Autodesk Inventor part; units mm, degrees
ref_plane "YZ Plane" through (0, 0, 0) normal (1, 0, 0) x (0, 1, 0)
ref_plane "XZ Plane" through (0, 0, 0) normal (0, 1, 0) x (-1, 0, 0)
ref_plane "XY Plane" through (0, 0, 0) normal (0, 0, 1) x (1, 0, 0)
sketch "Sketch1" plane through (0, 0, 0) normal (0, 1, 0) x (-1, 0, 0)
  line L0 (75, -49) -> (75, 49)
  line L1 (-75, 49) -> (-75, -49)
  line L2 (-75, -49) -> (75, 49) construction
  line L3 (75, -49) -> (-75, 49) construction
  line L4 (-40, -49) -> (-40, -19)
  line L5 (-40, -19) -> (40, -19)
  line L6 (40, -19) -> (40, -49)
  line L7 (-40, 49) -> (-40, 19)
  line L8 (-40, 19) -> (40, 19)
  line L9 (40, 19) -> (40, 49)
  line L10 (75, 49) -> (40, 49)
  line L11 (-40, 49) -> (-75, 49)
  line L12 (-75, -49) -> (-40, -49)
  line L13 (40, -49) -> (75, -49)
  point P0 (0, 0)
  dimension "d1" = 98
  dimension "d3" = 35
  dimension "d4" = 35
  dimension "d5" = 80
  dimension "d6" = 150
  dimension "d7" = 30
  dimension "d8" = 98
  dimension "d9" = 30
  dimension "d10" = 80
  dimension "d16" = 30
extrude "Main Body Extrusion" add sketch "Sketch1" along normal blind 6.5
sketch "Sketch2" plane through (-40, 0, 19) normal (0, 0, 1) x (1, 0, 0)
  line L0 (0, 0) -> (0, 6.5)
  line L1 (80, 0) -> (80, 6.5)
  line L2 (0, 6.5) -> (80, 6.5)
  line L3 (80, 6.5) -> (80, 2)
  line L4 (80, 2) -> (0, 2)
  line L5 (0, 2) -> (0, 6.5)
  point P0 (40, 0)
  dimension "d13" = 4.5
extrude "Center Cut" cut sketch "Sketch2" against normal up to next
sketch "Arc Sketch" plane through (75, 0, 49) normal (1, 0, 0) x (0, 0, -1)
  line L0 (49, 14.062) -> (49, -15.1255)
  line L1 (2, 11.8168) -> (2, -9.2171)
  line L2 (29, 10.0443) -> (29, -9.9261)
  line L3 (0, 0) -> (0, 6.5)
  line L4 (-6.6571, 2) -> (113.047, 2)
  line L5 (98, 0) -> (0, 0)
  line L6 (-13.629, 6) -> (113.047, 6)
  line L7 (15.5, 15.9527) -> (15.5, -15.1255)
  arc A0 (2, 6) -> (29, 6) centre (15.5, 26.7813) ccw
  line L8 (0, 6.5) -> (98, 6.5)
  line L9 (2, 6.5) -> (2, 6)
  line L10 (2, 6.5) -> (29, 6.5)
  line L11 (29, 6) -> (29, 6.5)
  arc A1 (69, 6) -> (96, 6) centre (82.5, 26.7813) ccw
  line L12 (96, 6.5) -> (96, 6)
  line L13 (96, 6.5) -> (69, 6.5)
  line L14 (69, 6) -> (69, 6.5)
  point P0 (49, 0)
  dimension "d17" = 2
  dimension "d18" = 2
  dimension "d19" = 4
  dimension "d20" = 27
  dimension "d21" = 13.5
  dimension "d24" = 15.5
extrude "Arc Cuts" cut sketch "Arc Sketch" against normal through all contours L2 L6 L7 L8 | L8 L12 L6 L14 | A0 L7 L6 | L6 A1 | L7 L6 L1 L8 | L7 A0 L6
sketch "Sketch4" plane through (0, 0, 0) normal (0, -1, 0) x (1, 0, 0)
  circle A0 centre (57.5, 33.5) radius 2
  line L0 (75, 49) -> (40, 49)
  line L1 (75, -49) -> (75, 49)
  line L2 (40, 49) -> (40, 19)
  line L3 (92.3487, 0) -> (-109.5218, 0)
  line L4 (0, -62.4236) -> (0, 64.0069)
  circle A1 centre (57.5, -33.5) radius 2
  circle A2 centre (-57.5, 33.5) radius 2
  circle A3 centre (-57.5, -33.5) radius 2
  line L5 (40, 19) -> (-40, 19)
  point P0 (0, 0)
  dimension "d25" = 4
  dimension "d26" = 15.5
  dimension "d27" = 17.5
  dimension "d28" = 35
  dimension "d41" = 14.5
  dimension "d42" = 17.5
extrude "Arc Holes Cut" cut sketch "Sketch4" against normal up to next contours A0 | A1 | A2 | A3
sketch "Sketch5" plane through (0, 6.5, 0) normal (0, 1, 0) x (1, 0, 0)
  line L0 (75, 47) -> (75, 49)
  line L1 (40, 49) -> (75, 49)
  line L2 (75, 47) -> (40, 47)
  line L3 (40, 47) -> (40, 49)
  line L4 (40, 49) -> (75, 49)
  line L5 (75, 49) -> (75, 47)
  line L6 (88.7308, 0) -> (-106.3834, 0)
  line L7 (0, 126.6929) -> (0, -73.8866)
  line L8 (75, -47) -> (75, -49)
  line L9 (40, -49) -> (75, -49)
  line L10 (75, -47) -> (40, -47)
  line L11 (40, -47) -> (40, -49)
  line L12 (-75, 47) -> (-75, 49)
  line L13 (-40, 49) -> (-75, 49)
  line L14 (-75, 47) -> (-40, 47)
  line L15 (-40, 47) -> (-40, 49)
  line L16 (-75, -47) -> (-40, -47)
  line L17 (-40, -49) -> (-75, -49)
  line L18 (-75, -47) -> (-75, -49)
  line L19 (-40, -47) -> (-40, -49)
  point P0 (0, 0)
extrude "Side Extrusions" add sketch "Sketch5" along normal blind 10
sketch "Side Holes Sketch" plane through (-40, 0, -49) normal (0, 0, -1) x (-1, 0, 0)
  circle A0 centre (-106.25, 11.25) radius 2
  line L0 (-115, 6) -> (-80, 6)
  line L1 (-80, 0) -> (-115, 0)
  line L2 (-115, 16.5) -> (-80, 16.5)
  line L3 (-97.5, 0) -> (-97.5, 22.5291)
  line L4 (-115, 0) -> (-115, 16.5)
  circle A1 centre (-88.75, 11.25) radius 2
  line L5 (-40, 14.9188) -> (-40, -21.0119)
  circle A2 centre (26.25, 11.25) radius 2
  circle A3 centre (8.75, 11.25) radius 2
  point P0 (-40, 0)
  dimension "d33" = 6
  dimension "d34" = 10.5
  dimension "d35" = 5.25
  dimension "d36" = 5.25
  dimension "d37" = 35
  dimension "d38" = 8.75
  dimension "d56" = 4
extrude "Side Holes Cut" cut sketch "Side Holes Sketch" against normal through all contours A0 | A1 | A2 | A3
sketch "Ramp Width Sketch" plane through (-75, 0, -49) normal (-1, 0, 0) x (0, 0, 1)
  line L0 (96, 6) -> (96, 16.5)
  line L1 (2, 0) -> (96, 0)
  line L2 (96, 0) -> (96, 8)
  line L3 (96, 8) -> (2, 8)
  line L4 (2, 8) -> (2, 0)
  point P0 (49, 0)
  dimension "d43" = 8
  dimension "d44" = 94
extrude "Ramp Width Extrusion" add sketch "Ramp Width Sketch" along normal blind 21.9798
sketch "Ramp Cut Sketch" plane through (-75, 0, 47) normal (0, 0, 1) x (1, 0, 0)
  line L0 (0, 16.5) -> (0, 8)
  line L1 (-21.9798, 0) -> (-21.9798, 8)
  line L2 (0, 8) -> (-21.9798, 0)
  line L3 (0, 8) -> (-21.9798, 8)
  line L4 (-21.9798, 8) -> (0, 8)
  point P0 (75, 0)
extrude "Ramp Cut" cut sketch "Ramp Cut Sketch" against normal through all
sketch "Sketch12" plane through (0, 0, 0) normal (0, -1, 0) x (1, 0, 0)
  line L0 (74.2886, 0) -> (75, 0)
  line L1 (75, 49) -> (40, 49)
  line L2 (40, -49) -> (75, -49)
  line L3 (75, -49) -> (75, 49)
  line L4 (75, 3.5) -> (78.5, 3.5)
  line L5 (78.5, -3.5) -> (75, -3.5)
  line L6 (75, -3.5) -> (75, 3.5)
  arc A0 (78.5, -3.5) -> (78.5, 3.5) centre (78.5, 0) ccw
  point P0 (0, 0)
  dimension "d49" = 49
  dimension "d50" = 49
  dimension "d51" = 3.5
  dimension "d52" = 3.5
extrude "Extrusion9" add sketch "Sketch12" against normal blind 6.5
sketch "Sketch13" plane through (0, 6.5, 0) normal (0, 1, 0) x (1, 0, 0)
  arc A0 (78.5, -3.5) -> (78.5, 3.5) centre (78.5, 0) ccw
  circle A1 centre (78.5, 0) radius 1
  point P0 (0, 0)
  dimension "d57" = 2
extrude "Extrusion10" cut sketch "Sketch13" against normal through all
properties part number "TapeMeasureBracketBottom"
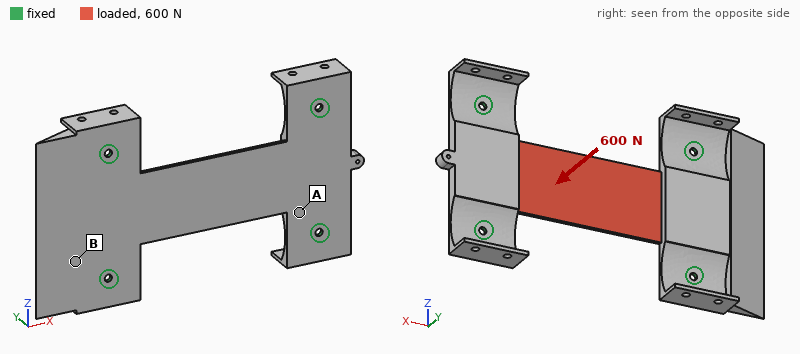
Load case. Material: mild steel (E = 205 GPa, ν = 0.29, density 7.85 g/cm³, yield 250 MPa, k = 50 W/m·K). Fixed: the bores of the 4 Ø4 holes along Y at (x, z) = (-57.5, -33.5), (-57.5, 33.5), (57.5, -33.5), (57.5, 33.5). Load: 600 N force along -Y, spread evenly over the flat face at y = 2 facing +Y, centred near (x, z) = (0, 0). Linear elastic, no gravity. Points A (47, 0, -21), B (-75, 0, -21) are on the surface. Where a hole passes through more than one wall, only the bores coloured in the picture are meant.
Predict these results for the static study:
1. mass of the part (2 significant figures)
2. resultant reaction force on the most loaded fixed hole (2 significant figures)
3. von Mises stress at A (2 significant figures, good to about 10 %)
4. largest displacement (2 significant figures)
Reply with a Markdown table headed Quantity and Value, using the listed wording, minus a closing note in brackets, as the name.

| Quantity | Value |
|---|---|
| mass of the part | 390 g |
| resultant reaction force on the most loaded fixed hole | 540 N |
| von Mises stress at A | 32 MPa |
| largest displacement | 0.30 mm |
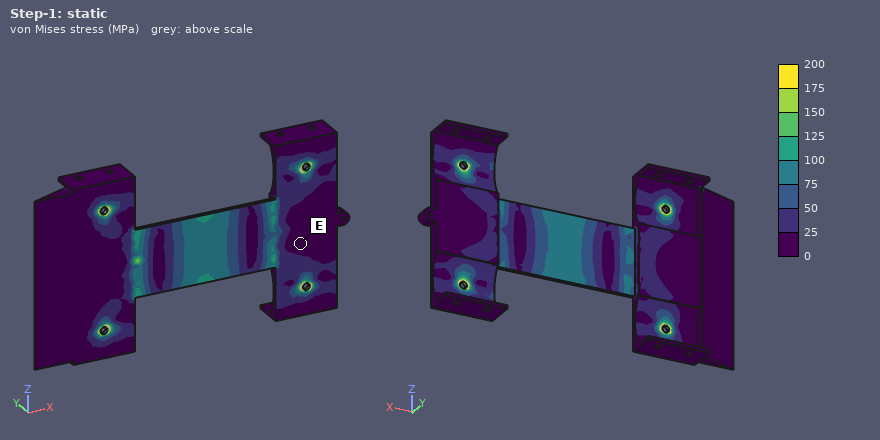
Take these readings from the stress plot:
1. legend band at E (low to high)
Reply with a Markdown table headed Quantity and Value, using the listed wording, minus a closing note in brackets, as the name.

| Quantity | Value |
|---|---|
| legend band at E | 0 to 25 MPa |
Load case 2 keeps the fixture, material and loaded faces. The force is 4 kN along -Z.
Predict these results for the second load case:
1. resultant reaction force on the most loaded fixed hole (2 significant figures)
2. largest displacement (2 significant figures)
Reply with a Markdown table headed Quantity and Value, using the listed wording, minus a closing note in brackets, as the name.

| Quantity | Value |
|---|---|
| resultant reaction force on the most loaded fixed hole | 1.3 kN |
| largest displacement | 63 µm |
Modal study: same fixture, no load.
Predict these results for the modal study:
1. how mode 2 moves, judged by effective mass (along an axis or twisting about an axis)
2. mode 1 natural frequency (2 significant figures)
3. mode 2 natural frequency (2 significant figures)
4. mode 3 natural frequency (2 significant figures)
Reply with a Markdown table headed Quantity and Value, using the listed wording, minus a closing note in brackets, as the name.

| Quantity | Value |
|---|---|
| how mode 2 moves, judged by effective mass | along Y |
| mode 1 natural frequency | 1000 Hz |
| mode 2 natural frequency | 1500 Hz |
| mode 3 natural frequency | 2400 Hz |
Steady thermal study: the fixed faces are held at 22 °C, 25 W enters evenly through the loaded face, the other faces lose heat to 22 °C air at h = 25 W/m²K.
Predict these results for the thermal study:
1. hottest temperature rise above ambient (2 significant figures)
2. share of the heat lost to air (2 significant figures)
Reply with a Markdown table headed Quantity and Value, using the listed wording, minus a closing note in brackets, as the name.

| Quantity | Value |
|---|---|
| hottest temperature rise above ambient | 78 K |
| share of the heat lost to air | 45 % |
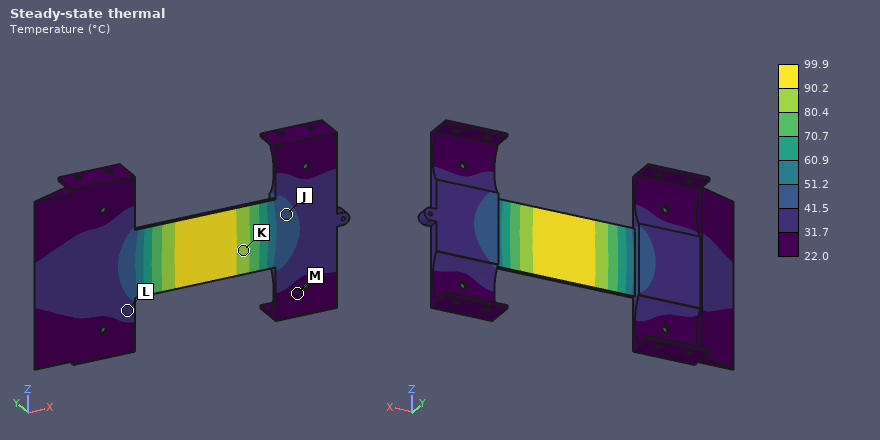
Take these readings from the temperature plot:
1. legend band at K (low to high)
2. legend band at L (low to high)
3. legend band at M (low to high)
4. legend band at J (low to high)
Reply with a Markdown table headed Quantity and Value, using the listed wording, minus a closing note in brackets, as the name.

| Quantity | Value |
|---|---|
| legend band at K | 80.4 to 90.2 °C |
| legend band at L | 31.7 to 41.5 °C |
| legend band at M | 22.0 to 31.7 °C |
| legend band at J | 41.5 to 51.2 °C |
